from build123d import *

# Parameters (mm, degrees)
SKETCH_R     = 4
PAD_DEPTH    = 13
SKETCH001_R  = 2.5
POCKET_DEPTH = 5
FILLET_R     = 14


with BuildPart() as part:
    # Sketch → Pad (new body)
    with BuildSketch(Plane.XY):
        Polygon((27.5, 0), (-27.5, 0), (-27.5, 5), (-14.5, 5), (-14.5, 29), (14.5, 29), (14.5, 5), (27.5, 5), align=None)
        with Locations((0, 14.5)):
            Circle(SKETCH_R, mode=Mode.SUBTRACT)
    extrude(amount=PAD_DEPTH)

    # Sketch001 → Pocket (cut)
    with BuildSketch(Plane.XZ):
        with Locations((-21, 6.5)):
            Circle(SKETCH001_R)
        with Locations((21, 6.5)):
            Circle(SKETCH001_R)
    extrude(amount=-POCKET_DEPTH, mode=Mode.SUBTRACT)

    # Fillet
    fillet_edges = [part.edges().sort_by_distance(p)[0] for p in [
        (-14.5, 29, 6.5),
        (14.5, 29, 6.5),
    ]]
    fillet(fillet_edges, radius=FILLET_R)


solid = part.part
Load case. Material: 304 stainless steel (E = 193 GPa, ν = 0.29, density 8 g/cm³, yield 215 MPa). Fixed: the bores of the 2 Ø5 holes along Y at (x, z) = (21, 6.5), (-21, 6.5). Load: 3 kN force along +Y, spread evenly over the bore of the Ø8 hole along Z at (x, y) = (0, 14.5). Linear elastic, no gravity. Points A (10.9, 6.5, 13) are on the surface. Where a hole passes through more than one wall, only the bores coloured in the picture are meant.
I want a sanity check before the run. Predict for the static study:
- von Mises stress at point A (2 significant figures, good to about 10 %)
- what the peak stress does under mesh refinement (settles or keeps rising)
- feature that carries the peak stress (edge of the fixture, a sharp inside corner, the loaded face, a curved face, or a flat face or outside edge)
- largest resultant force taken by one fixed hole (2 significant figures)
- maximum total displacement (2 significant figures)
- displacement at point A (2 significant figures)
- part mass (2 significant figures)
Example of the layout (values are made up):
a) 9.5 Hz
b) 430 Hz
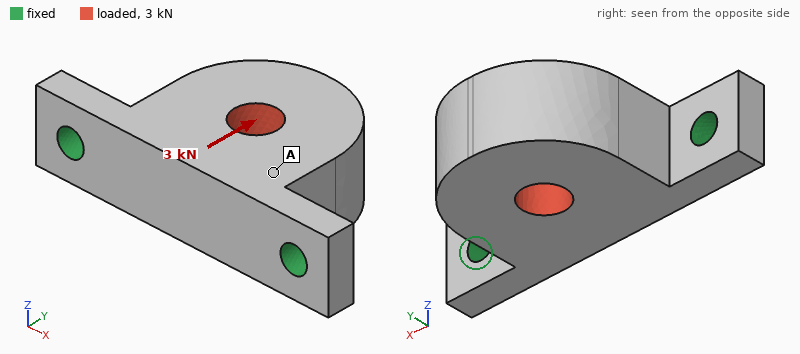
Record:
a) 23 MPa
b) keeps rising
c) edge of the fixture
d) 1.7 kN
e) 6.7 µm
f) 5.3 µm
g) 85 g
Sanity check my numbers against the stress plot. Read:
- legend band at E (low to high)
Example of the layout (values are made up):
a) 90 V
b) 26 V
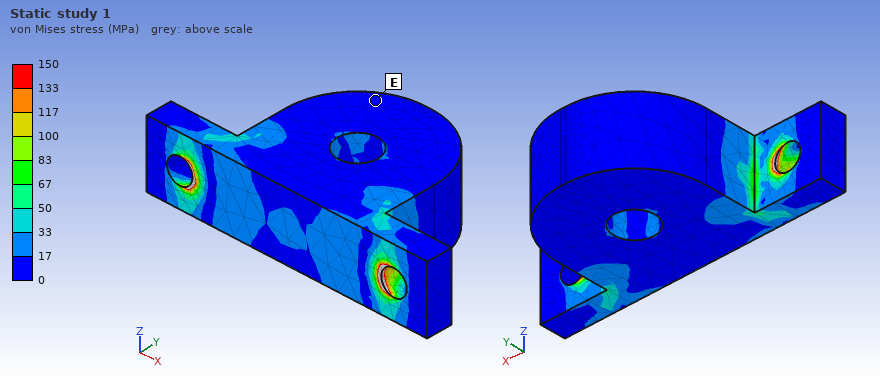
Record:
a) 0 to 17 MPa
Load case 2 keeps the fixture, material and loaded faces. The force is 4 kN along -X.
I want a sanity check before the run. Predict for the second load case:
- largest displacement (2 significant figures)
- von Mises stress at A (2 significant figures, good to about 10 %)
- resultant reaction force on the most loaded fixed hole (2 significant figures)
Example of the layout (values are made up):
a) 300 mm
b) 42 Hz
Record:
a) 10 µm
b) 33 MPa
c) 2.5 kN
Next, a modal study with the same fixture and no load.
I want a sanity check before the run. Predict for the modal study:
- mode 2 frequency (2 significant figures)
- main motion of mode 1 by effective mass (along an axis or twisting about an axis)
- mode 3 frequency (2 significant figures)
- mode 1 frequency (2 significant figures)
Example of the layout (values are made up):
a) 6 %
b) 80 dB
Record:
a) 13 kHz
b) along Z
c) 13 kHz
d) 4200 Hz
